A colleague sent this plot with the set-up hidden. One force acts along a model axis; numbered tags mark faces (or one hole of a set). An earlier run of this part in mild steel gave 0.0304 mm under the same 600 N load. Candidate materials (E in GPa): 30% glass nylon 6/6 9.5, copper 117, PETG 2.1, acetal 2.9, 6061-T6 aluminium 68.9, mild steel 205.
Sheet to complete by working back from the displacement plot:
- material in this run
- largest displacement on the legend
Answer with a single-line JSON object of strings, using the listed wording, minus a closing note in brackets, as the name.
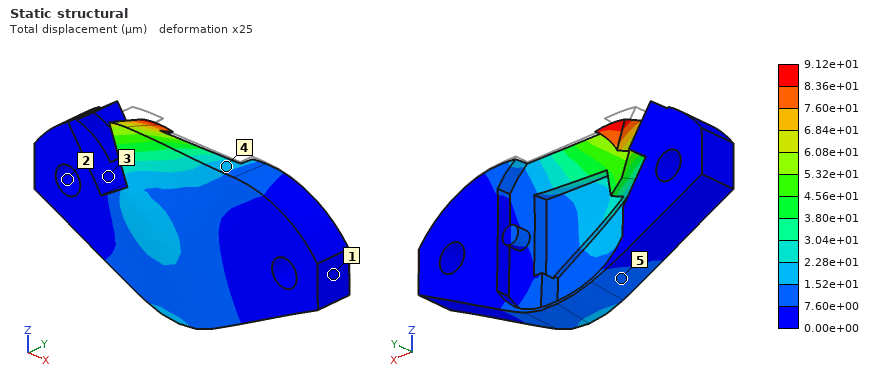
{"material in this run": "6061-T6 aluminium", "largest displacement on the legend": "9.12e+01 µm"}
